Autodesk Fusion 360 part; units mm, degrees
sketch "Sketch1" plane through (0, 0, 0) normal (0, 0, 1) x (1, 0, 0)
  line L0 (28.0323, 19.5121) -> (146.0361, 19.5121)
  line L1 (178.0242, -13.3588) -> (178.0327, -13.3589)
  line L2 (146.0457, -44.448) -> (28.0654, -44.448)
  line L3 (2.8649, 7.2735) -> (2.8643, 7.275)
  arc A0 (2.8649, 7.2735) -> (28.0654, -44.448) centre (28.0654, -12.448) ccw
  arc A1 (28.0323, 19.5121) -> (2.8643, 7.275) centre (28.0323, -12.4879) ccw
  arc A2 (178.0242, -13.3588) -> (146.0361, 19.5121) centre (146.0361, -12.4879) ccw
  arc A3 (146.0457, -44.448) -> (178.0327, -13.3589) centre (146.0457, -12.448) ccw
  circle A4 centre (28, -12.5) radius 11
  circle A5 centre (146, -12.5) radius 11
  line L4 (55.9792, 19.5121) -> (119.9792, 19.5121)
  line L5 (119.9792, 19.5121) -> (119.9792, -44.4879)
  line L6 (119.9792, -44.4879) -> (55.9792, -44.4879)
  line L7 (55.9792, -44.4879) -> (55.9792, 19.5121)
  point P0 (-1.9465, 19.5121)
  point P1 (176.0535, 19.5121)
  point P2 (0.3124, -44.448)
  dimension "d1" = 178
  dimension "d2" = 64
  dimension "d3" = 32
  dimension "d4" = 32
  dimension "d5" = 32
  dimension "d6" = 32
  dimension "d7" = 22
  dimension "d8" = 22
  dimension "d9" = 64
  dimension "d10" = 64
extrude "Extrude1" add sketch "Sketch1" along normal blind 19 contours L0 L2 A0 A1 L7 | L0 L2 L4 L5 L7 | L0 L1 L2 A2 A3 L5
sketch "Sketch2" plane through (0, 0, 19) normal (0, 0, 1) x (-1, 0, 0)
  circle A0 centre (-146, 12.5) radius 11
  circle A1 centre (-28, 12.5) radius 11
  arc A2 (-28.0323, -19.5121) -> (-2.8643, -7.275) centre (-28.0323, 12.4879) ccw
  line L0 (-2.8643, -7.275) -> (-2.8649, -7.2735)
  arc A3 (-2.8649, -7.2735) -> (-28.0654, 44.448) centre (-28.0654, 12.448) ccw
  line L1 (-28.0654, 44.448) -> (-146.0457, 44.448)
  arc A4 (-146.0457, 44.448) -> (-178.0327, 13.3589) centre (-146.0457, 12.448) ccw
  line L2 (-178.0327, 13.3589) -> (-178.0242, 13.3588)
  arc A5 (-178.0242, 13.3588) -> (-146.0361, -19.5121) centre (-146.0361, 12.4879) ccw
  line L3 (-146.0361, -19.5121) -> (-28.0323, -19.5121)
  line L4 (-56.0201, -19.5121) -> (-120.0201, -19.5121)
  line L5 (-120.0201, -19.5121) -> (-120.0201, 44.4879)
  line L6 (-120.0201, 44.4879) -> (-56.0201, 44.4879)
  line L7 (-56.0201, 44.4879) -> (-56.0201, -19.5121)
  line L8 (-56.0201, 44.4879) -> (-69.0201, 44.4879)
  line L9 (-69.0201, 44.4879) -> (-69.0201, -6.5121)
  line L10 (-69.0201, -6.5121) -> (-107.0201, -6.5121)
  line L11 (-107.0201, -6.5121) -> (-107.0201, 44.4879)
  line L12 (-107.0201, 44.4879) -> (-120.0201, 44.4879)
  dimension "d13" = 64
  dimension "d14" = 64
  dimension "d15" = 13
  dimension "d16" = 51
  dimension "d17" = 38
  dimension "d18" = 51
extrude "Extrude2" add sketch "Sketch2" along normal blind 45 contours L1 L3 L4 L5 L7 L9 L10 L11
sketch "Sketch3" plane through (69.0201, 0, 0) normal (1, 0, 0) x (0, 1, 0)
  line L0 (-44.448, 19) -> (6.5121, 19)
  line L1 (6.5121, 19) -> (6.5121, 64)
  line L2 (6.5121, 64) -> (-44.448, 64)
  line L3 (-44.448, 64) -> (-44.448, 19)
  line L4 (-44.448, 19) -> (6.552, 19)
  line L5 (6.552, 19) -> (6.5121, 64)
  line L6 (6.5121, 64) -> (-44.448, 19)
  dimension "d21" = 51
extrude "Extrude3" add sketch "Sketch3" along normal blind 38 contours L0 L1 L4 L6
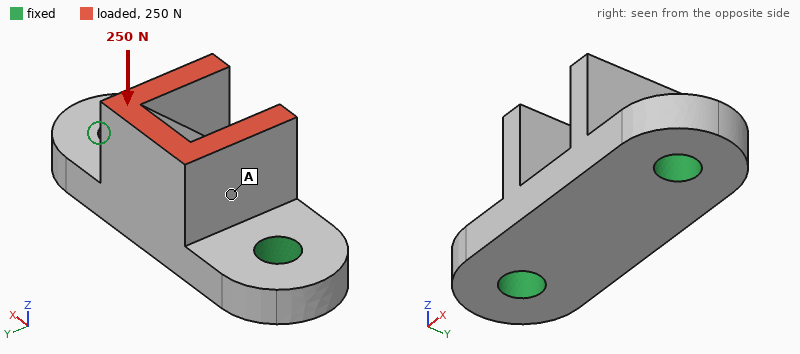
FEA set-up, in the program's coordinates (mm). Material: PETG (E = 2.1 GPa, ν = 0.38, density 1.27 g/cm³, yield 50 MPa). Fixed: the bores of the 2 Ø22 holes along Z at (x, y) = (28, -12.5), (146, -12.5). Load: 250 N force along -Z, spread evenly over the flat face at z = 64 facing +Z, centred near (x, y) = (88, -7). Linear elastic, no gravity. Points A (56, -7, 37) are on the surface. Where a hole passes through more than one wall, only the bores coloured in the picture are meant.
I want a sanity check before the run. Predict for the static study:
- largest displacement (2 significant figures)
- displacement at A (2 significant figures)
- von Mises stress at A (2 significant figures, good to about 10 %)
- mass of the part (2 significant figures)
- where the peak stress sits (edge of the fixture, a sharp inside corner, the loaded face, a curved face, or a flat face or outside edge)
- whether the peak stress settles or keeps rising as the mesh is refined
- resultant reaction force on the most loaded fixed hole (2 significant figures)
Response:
19 µm
11 µm
0.15 MPa
420 g
edge of the fixture
keeps rising
130 N
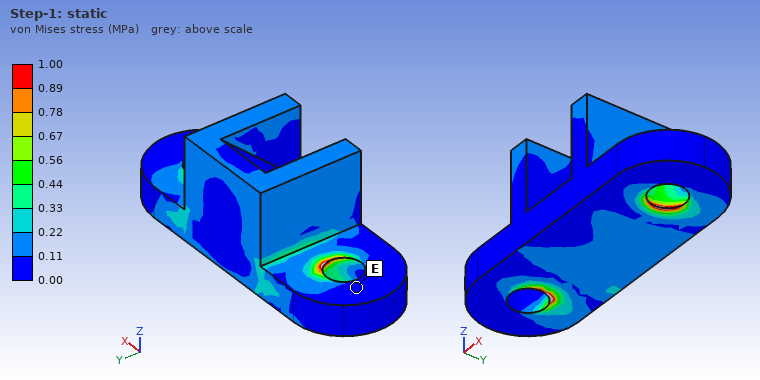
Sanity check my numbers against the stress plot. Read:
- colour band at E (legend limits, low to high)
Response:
0.00 to 0.11 MPa
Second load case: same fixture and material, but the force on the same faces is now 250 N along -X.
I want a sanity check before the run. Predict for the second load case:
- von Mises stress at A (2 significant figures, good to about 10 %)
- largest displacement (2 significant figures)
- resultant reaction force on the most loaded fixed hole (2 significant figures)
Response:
0.44 MPa
59 µm
200 N
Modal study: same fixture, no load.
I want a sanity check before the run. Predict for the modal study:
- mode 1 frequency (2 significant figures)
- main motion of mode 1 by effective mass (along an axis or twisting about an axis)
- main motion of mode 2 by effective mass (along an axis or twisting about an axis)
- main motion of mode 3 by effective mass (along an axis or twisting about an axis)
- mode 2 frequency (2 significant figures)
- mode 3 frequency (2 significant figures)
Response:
850 Hz
along Y
along Z
along X
1500 Hz
1800 Hz
